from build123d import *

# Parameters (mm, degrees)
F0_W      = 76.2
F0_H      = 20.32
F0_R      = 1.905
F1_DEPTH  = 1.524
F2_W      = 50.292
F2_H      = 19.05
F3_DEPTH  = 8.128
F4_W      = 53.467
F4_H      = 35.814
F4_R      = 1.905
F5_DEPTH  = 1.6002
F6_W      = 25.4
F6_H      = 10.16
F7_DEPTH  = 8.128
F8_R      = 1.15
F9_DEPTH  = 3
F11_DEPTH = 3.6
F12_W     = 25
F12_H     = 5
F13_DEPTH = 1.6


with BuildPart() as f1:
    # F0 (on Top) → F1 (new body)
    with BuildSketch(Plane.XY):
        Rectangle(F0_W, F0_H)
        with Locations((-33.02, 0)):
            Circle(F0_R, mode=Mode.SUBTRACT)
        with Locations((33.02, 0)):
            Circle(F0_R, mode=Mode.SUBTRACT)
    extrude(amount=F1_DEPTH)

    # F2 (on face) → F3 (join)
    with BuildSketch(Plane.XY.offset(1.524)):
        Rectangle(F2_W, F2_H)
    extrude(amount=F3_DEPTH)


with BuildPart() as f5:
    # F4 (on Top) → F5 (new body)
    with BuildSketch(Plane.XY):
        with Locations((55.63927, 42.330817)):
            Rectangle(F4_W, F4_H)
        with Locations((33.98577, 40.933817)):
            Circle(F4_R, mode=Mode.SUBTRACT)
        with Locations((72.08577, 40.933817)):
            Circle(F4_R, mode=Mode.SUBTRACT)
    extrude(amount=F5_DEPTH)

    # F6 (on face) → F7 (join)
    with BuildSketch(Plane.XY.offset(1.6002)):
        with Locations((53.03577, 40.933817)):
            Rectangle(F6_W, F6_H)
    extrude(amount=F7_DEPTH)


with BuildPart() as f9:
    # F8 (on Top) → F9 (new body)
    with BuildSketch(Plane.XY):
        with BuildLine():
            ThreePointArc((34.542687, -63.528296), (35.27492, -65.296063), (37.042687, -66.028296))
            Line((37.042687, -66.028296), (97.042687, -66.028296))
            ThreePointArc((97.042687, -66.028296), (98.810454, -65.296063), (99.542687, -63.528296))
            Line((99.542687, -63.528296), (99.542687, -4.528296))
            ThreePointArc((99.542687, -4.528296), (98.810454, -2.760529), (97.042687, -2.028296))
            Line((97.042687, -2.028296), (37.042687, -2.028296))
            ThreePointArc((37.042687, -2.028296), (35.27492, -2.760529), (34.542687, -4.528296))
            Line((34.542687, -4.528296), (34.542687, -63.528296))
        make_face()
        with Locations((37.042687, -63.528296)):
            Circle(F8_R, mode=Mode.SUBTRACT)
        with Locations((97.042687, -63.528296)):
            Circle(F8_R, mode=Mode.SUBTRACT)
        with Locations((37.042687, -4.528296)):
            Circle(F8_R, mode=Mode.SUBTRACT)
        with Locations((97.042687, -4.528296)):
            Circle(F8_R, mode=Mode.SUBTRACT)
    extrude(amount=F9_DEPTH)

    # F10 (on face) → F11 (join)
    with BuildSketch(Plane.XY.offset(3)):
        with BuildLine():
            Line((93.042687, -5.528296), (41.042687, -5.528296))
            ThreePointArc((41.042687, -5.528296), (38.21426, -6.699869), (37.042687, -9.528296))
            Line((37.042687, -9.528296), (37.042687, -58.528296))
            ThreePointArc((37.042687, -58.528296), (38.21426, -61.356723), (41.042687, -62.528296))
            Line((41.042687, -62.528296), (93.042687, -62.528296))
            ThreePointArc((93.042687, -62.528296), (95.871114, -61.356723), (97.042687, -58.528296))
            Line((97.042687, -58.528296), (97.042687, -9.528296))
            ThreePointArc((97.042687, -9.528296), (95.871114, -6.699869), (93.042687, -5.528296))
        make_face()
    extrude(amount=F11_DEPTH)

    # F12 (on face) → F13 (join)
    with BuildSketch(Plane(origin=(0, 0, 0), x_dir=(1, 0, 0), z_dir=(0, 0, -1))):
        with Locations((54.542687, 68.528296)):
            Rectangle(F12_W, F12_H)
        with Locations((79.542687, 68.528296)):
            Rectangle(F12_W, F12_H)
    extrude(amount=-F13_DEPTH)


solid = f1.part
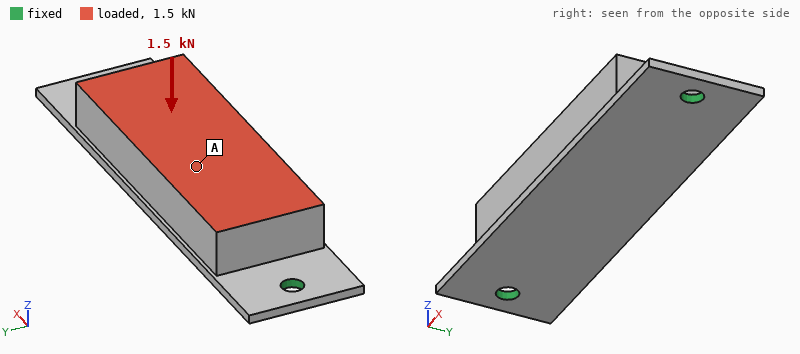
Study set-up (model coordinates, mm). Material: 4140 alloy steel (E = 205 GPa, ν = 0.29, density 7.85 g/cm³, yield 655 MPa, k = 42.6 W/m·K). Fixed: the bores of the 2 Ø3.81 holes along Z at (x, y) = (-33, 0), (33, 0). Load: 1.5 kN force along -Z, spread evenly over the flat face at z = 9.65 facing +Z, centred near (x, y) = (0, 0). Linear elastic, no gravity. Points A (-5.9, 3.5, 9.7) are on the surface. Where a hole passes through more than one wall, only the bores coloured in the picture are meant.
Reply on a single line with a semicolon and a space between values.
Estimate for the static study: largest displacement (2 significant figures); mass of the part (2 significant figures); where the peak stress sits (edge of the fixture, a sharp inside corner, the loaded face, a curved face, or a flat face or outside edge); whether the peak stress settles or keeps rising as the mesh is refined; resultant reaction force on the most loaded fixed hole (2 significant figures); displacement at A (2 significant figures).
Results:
45 µm; 79 g; edge of the fixture; keeps rising; 1.1 kN; 44 µm
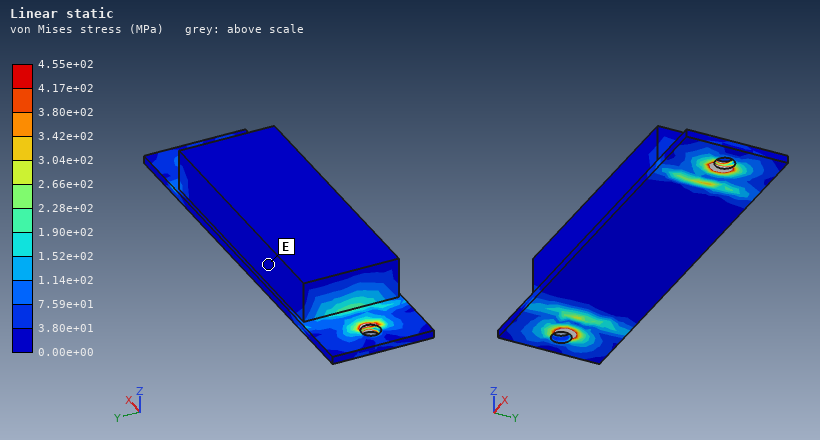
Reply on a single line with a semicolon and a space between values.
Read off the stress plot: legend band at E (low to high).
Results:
0.00e+00 to 3.80e+01 MPa
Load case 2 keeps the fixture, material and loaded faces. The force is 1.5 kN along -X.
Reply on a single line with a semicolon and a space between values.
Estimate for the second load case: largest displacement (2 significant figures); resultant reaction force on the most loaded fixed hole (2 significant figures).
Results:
10 µm; 780 N
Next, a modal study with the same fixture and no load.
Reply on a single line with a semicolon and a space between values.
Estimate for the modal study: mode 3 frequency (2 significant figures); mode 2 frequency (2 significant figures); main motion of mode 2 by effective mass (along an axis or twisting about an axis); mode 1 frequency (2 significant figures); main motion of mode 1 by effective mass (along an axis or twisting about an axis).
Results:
6800 Hz; 3500 Hz; along Z; 2200 Hz; along Y
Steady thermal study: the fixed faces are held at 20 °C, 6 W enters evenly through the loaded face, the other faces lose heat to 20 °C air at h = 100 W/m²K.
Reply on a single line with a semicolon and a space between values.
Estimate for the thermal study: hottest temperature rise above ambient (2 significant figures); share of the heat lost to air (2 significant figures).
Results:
15 K; 58 %
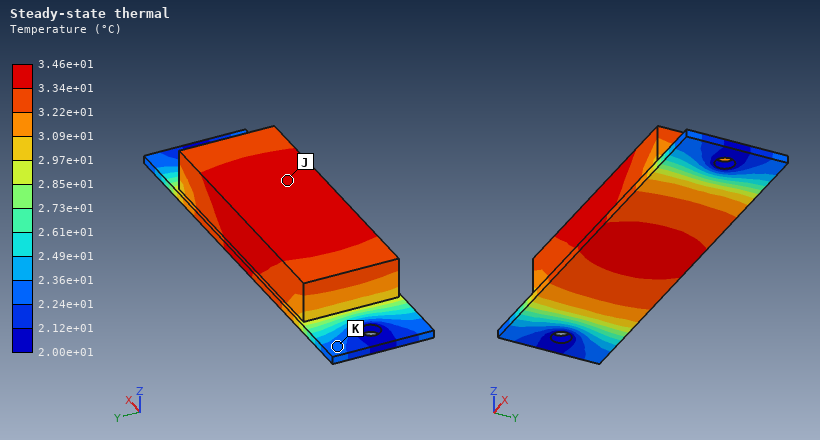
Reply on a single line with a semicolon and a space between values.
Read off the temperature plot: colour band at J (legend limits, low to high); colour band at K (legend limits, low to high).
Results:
3.34e+01 to 3.46e+01 °C; 2.24e+01 to 2.36e+01 °C
